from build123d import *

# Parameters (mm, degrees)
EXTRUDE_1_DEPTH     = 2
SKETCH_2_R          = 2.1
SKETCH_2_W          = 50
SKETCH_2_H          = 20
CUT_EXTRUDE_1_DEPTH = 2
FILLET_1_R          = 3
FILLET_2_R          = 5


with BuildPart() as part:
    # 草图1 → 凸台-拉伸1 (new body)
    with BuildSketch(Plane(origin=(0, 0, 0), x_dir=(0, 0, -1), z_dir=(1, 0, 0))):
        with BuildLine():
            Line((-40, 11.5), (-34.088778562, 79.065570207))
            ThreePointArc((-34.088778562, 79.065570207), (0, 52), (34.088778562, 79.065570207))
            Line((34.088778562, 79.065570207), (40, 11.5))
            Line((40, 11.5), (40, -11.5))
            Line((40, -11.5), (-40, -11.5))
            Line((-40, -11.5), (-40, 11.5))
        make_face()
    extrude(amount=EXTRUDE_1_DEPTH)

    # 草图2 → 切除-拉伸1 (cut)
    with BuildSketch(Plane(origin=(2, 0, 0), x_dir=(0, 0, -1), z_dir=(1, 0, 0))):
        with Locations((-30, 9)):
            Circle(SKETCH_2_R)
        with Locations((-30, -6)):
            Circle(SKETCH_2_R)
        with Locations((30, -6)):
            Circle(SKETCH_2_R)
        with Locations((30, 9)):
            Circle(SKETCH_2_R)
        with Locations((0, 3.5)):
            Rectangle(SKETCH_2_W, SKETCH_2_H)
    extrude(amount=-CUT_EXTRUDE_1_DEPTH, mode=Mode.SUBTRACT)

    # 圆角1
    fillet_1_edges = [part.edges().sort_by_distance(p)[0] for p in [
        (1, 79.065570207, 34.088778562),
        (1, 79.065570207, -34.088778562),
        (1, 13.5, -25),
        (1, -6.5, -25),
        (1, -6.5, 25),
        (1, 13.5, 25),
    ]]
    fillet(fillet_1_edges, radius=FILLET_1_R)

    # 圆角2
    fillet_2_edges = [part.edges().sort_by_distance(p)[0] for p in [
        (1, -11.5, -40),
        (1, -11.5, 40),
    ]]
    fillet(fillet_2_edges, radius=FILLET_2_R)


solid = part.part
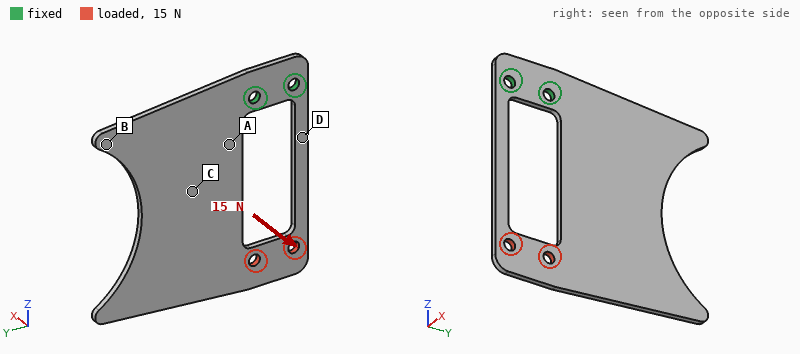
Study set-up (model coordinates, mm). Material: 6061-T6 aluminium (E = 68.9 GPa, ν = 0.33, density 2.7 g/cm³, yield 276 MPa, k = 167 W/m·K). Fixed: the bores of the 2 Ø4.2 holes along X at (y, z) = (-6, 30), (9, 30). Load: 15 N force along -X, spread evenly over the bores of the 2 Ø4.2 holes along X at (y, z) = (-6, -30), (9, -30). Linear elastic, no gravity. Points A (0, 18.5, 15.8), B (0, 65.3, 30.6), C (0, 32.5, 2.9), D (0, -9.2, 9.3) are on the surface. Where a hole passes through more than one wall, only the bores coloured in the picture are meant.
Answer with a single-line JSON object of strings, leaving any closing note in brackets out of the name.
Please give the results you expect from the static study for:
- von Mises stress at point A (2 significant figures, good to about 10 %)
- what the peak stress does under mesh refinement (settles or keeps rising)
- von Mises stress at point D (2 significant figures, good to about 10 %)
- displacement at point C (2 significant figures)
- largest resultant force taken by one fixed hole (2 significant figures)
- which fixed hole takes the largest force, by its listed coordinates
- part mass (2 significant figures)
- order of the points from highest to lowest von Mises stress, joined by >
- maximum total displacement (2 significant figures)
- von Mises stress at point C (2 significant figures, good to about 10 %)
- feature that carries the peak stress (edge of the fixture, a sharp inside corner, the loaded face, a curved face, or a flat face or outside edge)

{"von Mises stress at point A": "30 MPa", "what the peak stress does under mesh refinement": "keeps rising", "von Mises stress at point D": "43 MPa", "displacement at point C": "0.27 mm", "largest resultant force taken by one fixed hole": "11 N", "which fixed hole takes the largest force, by its listed coordinates": "(-6, 30)", "part mass": "24 g", "order of the points from highest to lowest von Mises stress, joined by >": "D > A > C > B", "maximum total displacement": "1.2 mm", "von Mises stress at point C": "16 MPa", "feature that carries the peak stress": "edge of the fixture"}
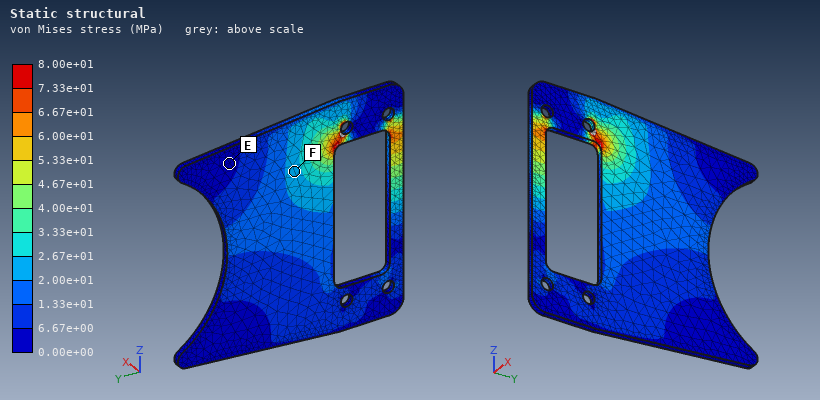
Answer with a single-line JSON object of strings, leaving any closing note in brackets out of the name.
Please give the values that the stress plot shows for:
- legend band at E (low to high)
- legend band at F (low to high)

{"legend band at E": "0.00e+00 to 6.67e+00 MPa", "legend band at F": "2.00e+01 to 2.67e+01 MPa"}
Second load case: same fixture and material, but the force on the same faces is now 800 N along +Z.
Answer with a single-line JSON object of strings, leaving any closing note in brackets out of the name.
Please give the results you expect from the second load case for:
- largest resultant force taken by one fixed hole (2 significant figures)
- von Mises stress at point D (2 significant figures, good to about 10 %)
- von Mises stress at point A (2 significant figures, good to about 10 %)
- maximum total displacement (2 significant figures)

{"largest resultant force taken by one fixed hole": "400 N", "von Mises stress at point D": "41 MPa", "von Mises stress at point A": "18 MPa", "maximum total displacement": "43 µm"}
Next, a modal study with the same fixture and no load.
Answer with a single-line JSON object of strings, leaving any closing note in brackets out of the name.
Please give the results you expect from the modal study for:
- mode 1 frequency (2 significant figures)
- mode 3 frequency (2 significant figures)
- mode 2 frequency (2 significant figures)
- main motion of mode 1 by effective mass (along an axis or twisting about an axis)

{"mode 1 frequency": "200 Hz", "mode 3 frequency": "930 Hz", "mode 2 frequency": "420 Hz", "main motion of mode 1 by effective mass": "along X"}
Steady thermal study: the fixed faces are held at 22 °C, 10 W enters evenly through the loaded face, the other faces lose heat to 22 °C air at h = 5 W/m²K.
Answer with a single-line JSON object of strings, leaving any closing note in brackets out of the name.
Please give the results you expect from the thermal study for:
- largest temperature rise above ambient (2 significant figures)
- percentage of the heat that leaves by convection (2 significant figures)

{"largest temperature rise above ambient": "76 K", "percentage of the heat that leaves by convection": "15 %"}
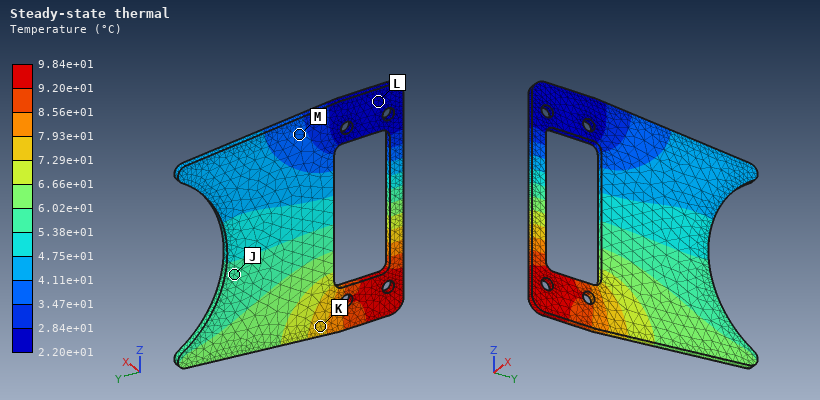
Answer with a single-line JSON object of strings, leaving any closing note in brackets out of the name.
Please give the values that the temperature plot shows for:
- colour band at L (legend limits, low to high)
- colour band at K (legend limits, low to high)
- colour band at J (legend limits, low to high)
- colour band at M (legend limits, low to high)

{"colour band at L": "2.20e+01 to 2.84e+01 °C", "colour band at K": "7.29e+01 to 7.93e+01 °C", "colour band at J": "5.38e+01 to 6.02e+01 °C", "colour band at M": "3.47e+01 to 4.11e+01 °C"}
